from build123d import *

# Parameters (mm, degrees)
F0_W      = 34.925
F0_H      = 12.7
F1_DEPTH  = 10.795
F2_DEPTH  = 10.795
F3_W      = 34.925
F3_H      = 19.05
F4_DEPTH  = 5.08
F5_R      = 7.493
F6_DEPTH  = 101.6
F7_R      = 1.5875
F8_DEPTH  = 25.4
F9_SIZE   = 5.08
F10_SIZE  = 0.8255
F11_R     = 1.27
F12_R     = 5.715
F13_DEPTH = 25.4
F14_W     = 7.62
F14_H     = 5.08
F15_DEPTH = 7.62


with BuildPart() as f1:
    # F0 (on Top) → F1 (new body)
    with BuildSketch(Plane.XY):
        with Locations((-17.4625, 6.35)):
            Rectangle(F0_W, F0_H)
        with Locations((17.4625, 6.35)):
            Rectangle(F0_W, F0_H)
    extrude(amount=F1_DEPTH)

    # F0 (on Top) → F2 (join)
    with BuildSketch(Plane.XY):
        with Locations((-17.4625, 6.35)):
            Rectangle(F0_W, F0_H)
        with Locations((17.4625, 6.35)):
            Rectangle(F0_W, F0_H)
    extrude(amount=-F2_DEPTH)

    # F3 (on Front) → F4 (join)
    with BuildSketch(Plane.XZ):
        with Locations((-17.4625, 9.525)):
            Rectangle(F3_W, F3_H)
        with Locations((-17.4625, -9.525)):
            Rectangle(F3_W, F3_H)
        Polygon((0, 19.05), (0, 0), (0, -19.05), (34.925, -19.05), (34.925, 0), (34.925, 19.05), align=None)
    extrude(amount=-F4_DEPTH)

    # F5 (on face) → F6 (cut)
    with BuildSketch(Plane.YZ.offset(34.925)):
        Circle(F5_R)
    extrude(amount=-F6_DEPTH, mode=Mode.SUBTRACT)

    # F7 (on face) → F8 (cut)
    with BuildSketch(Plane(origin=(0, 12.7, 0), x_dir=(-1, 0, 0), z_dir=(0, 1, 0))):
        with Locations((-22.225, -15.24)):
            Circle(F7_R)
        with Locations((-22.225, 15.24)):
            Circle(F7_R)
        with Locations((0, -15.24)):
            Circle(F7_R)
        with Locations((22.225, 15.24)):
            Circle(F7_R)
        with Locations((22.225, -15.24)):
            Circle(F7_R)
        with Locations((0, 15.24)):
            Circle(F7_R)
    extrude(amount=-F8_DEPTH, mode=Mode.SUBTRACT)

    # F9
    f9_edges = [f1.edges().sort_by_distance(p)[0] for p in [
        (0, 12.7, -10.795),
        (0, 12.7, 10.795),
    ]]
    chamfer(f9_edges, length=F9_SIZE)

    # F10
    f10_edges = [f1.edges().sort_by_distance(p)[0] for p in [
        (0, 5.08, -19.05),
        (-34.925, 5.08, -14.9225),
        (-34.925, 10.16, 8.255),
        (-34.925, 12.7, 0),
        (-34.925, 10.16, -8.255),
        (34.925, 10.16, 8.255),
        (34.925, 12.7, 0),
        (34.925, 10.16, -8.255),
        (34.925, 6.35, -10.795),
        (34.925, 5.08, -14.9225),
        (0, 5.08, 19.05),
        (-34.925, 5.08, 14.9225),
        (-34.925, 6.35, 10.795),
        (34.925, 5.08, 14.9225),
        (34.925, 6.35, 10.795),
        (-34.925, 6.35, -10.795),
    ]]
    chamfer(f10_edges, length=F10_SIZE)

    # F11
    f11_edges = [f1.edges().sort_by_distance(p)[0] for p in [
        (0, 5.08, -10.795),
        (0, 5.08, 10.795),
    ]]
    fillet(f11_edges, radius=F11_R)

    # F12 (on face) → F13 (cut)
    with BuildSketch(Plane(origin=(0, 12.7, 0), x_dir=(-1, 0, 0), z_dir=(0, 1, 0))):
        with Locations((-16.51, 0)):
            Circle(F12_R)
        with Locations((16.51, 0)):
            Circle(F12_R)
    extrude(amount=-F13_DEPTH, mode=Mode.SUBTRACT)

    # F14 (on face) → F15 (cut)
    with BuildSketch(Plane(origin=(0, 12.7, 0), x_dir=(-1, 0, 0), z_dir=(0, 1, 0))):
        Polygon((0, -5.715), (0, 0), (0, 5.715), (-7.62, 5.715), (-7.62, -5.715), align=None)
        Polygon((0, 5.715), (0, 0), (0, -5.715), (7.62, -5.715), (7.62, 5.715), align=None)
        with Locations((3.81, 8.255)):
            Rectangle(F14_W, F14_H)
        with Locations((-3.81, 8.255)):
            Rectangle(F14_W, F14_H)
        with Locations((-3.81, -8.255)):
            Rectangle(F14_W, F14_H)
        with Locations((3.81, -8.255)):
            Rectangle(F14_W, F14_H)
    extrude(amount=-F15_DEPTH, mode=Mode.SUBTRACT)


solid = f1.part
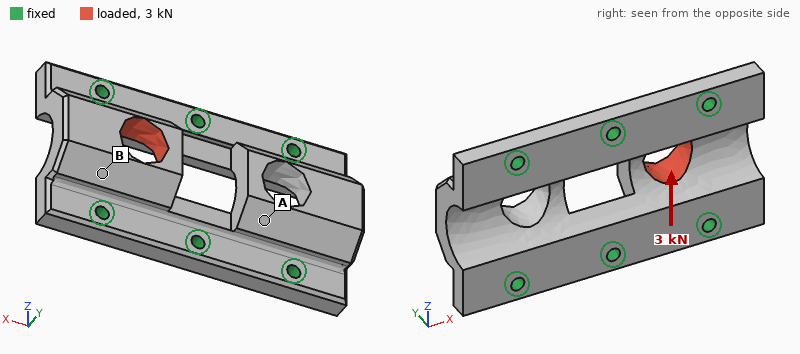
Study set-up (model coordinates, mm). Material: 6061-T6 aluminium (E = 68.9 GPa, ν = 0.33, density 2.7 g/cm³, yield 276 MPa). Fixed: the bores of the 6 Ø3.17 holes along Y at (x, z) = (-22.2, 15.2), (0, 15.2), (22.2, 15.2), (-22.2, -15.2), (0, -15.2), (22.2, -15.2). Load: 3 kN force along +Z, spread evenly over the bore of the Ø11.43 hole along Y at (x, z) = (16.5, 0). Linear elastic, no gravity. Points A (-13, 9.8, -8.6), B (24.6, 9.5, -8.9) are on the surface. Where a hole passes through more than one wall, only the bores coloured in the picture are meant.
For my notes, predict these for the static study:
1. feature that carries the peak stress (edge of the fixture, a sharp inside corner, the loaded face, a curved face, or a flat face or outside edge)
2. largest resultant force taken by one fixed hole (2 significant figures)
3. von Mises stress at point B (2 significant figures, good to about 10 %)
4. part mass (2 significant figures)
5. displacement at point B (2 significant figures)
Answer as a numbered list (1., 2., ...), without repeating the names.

1. a curved face
2. 1.3 kN
3. 14 MPa
4. 37 g
5. 6.2 µm
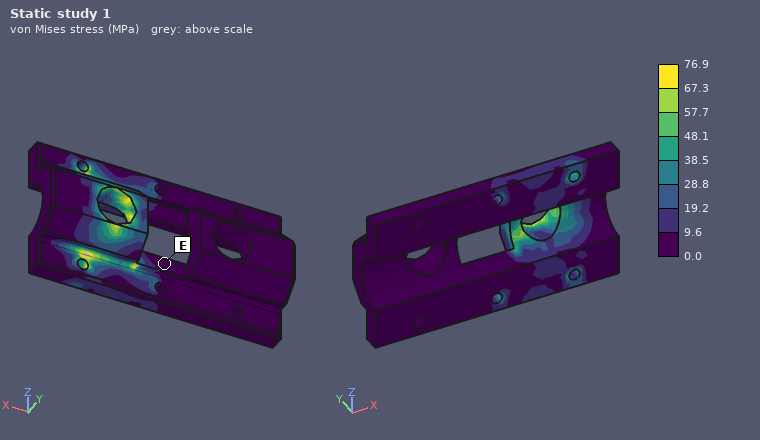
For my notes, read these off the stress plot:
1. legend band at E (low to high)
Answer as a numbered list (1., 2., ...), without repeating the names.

1. 0.0 to 9.6 MPa
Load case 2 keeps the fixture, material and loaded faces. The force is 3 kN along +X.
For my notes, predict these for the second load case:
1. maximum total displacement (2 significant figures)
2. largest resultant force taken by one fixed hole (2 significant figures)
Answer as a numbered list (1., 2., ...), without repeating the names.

1. 25 µm
2. 1.0 kN
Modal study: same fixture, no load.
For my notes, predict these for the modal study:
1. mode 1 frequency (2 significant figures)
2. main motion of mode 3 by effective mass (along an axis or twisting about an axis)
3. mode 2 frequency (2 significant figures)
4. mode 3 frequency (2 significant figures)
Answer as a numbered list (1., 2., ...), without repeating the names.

1. 17 kHz
2. along Y
3. 17 kHz
4. 27 kHz
